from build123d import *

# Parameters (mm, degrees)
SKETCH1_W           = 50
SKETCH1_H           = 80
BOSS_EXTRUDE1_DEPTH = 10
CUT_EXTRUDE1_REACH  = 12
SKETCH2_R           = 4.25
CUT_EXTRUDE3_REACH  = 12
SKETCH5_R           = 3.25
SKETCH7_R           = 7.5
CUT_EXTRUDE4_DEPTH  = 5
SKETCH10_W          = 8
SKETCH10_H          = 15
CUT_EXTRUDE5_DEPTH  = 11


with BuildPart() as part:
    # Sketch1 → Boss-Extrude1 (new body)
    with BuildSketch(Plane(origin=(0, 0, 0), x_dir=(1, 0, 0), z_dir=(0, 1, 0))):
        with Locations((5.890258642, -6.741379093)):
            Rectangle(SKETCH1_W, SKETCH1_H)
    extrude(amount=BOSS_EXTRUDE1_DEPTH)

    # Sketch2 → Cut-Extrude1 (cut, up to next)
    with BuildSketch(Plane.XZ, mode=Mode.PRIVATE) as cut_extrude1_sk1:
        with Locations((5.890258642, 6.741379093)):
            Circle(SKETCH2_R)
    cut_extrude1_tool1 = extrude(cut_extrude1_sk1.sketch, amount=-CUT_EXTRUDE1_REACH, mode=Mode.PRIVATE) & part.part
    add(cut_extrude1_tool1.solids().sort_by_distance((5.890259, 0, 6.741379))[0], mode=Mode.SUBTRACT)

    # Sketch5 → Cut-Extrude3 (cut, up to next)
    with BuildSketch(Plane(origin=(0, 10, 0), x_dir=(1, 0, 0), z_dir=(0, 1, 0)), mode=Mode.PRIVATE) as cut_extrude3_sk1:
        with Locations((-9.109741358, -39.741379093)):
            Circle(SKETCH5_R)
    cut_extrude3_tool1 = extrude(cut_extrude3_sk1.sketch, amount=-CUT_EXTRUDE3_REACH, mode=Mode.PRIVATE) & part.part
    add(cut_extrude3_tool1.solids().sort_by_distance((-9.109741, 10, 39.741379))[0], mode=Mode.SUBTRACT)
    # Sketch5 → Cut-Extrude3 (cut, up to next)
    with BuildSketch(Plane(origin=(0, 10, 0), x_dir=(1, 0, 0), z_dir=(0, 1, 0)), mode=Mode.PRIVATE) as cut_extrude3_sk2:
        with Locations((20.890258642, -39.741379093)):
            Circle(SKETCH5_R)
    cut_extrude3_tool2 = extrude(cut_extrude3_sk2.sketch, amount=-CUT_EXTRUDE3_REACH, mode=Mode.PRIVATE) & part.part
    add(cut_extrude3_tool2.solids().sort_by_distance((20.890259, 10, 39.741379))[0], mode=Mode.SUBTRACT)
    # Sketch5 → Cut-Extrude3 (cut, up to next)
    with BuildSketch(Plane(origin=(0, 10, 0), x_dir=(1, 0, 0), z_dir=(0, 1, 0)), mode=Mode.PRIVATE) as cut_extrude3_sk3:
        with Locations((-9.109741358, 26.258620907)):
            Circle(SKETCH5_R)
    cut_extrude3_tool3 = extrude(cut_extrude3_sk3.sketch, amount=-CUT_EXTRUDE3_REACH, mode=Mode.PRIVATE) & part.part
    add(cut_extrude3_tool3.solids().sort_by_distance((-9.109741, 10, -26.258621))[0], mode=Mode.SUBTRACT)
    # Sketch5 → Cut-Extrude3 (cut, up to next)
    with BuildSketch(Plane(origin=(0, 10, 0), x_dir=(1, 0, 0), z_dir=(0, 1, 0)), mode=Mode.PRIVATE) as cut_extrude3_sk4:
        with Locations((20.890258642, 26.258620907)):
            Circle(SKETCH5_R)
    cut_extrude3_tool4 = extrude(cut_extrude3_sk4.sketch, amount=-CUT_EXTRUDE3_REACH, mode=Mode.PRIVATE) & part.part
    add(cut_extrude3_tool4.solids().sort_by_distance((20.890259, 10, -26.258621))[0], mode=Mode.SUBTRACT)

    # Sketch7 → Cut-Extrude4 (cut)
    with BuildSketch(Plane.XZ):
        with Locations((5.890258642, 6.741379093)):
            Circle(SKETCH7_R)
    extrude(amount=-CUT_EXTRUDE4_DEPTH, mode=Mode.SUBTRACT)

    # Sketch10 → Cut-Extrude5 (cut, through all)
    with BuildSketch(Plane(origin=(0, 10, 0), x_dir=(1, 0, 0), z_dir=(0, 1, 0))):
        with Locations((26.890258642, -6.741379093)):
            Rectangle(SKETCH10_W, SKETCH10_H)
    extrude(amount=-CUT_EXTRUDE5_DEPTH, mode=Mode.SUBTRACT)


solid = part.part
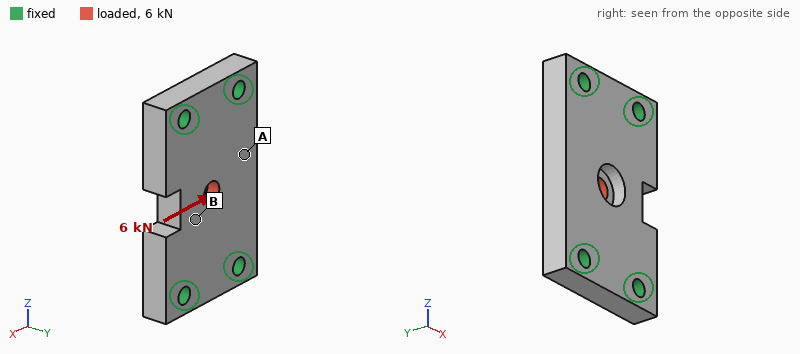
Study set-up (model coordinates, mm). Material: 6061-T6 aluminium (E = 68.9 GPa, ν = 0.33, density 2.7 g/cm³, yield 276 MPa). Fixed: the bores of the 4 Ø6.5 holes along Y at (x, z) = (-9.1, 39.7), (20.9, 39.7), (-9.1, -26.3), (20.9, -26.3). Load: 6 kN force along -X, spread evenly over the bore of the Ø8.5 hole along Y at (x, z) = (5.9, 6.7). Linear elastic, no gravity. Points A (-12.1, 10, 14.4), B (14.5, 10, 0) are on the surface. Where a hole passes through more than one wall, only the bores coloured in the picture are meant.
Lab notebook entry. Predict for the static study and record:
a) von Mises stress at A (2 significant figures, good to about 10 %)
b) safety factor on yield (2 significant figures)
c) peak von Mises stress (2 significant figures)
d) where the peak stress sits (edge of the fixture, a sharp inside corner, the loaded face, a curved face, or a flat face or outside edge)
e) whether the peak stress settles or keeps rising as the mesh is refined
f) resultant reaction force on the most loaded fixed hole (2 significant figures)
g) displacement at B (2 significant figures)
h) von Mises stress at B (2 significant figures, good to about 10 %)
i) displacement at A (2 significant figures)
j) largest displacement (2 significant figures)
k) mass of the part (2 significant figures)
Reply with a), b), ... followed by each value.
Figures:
a) 12 MPa
b) 3.4
c) 80 MPa
d) the loaded face
e) settles
f) 2.2 kN
g) 11 µm
h) 30 MPa
i) 10.0 µm
j) 16 µm
k) 98 g
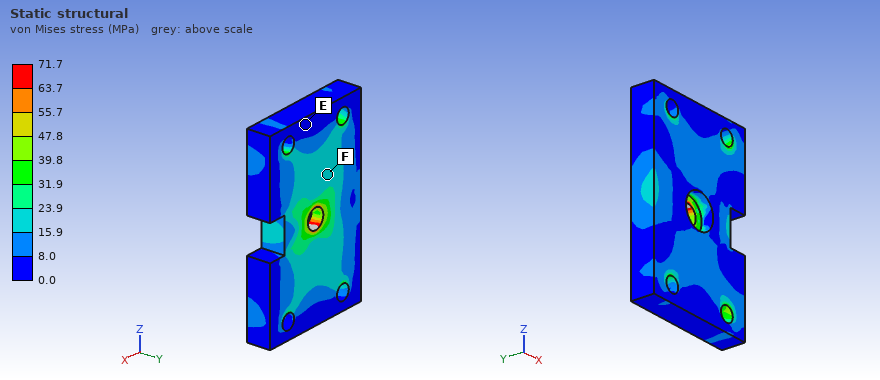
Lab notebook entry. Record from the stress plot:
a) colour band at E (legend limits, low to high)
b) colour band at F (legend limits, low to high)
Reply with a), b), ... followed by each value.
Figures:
a) 0.0 to 8.0 MPa
b) 15.9 to 23.9 MPa
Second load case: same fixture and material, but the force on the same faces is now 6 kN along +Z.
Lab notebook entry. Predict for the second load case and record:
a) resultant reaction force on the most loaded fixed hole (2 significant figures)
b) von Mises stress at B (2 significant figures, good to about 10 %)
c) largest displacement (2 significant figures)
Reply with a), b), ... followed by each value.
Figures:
a) 1.6 kN
b) 16 MPa
c) 8.7 µm
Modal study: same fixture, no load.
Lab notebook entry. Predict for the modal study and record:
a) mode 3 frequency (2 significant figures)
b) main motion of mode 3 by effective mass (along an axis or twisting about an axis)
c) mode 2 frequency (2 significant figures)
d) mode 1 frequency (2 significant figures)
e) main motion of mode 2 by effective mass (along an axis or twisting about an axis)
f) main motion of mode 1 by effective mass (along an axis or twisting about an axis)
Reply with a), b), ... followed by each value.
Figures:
a) 21 kHz
b) along X
c) 14 kHz
d) 11 kHz
e) twisting about Z
f) along Y
